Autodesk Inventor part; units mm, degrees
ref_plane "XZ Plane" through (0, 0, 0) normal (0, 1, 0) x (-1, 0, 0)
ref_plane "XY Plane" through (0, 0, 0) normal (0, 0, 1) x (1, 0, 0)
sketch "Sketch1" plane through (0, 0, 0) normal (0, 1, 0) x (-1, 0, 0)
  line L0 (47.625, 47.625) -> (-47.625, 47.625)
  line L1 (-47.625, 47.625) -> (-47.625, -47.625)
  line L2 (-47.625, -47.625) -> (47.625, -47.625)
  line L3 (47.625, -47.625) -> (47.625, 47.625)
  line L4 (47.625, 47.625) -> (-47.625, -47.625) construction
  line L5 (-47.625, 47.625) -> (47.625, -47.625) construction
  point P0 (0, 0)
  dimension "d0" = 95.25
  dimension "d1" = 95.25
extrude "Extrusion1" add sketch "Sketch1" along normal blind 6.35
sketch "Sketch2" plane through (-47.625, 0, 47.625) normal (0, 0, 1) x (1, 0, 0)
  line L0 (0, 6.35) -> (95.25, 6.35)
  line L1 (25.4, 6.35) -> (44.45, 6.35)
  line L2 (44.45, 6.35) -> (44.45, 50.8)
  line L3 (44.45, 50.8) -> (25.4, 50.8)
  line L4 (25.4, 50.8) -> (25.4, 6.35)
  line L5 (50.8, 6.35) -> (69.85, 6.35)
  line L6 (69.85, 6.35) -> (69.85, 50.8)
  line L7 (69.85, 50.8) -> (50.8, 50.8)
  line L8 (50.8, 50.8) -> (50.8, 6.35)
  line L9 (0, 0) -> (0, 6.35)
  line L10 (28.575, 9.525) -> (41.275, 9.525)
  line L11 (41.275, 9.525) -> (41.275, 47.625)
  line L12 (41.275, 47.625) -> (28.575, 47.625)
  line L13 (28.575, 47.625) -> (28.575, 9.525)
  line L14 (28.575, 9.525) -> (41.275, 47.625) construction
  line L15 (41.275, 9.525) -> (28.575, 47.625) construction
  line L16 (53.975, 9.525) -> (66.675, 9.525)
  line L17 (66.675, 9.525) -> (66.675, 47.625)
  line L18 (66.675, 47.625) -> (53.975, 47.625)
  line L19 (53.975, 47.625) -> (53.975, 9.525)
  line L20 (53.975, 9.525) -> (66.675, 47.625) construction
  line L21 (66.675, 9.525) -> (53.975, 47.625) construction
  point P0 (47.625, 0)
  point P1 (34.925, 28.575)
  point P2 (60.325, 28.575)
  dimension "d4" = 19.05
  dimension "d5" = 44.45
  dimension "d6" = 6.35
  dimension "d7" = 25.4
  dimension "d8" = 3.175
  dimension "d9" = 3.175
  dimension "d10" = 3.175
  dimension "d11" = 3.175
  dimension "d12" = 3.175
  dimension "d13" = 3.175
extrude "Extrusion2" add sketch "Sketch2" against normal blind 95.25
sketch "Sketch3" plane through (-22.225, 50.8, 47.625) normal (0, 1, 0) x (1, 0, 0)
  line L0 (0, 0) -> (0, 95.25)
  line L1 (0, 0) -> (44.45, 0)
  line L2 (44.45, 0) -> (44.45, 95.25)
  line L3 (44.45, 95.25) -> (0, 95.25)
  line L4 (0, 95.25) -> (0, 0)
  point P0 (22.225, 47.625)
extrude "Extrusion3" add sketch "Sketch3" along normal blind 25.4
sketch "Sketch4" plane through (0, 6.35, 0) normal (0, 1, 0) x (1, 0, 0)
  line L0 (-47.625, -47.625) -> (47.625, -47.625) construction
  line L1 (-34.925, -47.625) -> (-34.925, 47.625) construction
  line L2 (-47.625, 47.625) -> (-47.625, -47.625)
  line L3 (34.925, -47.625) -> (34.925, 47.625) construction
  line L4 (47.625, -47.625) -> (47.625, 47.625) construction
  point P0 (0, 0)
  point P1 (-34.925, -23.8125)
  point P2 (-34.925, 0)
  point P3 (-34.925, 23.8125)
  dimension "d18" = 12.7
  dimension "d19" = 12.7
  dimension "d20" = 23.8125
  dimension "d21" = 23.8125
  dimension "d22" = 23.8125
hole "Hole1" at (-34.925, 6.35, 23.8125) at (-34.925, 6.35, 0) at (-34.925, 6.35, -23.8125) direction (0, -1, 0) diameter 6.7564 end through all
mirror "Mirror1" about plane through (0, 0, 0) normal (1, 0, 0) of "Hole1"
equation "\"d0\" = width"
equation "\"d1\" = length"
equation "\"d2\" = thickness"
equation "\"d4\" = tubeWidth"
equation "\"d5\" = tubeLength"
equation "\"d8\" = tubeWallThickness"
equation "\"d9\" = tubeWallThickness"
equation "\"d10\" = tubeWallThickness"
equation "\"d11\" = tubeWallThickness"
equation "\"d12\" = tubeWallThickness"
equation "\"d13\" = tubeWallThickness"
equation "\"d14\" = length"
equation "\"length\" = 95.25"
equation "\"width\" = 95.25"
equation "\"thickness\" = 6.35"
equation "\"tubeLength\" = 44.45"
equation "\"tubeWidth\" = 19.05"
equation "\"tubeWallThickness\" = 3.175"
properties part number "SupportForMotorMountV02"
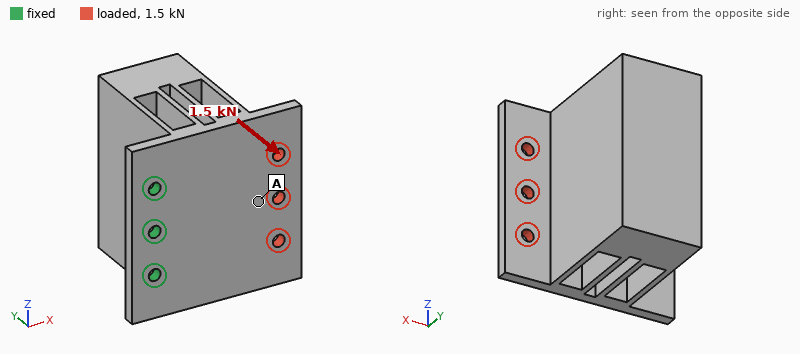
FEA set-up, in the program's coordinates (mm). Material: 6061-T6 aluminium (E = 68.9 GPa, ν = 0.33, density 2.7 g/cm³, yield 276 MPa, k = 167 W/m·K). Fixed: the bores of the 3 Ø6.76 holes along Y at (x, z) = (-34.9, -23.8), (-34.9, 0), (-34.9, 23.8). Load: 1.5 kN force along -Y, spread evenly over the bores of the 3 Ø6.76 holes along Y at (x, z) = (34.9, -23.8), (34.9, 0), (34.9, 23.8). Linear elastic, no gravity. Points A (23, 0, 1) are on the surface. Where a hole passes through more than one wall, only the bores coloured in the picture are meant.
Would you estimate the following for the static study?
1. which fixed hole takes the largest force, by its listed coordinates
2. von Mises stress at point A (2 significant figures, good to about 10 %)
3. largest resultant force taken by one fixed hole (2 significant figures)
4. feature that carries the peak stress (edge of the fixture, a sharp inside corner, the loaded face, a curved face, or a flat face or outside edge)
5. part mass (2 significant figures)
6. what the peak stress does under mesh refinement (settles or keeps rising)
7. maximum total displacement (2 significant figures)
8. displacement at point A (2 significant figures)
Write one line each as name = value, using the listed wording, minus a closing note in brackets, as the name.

which fixed hole takes the largest force, by its listed coordinates = (-34.9, 0)
von Mises stress at point A = 28 MPa
largest resultant force taken by one fixed hole = 780 N
feature that carries the peak stress = edge of the fixture
part mass = 630 g
what the peak stress does under mesh refinement = keeps rising
maximum total displacement = 0.99 mm
displacement at point A = 0.57 mm
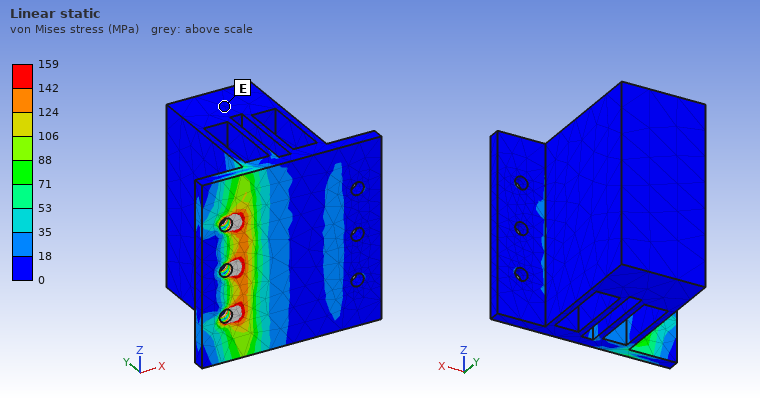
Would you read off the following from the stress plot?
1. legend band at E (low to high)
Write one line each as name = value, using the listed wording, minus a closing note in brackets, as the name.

legend band at E = 0 to 18 MPa
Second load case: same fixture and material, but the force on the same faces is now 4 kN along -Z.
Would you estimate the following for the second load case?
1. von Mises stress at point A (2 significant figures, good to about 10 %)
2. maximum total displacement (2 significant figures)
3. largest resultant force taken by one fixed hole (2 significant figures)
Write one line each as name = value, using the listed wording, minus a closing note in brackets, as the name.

von Mises stress at point A = 18 MPa
maximum total displacement = 68 µm
largest resultant force taken by one fixed hole = 5.4 kN
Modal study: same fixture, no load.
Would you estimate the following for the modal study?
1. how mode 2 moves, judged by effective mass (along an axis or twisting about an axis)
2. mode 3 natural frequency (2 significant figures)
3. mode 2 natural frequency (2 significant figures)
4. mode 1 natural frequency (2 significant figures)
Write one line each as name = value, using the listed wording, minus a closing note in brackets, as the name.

how mode 2 moves, judged by effective mass = along Z
mode 3 natural frequency = 1600 Hz
mode 2 natural frequency = 1100 Hz
mode 1 natural frequency = 320 Hz
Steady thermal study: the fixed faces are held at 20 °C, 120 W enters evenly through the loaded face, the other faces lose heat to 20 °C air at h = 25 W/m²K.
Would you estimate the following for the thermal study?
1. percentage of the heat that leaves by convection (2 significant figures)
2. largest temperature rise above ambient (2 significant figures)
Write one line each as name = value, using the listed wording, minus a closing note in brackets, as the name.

percentage of the heat that leaves by convection = 33 %
largest temperature rise above ambient = 66 K
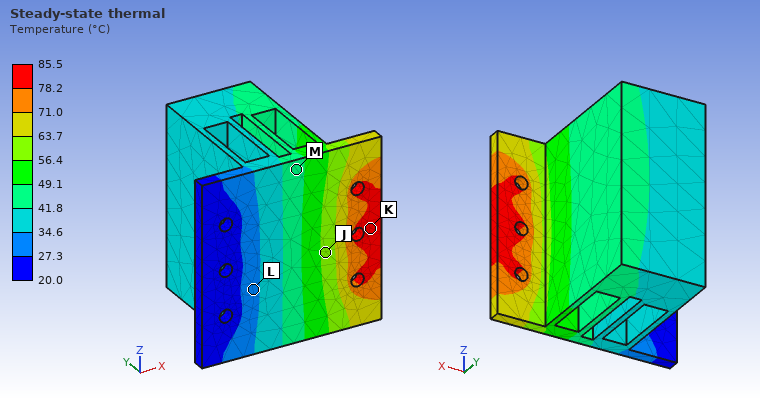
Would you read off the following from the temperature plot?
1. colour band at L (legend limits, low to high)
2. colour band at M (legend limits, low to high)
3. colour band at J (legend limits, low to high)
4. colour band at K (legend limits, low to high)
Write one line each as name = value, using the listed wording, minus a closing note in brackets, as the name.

colour band at L = 27.3 to 34.6 °C
colour band at M = 41.8 to 49.1 °C
colour band at J = 56.4 to 63.7 °C
colour band at K = 78.2 to 85.5 °C
